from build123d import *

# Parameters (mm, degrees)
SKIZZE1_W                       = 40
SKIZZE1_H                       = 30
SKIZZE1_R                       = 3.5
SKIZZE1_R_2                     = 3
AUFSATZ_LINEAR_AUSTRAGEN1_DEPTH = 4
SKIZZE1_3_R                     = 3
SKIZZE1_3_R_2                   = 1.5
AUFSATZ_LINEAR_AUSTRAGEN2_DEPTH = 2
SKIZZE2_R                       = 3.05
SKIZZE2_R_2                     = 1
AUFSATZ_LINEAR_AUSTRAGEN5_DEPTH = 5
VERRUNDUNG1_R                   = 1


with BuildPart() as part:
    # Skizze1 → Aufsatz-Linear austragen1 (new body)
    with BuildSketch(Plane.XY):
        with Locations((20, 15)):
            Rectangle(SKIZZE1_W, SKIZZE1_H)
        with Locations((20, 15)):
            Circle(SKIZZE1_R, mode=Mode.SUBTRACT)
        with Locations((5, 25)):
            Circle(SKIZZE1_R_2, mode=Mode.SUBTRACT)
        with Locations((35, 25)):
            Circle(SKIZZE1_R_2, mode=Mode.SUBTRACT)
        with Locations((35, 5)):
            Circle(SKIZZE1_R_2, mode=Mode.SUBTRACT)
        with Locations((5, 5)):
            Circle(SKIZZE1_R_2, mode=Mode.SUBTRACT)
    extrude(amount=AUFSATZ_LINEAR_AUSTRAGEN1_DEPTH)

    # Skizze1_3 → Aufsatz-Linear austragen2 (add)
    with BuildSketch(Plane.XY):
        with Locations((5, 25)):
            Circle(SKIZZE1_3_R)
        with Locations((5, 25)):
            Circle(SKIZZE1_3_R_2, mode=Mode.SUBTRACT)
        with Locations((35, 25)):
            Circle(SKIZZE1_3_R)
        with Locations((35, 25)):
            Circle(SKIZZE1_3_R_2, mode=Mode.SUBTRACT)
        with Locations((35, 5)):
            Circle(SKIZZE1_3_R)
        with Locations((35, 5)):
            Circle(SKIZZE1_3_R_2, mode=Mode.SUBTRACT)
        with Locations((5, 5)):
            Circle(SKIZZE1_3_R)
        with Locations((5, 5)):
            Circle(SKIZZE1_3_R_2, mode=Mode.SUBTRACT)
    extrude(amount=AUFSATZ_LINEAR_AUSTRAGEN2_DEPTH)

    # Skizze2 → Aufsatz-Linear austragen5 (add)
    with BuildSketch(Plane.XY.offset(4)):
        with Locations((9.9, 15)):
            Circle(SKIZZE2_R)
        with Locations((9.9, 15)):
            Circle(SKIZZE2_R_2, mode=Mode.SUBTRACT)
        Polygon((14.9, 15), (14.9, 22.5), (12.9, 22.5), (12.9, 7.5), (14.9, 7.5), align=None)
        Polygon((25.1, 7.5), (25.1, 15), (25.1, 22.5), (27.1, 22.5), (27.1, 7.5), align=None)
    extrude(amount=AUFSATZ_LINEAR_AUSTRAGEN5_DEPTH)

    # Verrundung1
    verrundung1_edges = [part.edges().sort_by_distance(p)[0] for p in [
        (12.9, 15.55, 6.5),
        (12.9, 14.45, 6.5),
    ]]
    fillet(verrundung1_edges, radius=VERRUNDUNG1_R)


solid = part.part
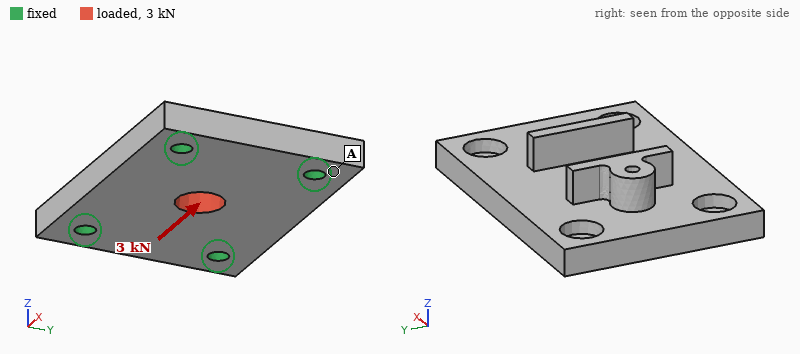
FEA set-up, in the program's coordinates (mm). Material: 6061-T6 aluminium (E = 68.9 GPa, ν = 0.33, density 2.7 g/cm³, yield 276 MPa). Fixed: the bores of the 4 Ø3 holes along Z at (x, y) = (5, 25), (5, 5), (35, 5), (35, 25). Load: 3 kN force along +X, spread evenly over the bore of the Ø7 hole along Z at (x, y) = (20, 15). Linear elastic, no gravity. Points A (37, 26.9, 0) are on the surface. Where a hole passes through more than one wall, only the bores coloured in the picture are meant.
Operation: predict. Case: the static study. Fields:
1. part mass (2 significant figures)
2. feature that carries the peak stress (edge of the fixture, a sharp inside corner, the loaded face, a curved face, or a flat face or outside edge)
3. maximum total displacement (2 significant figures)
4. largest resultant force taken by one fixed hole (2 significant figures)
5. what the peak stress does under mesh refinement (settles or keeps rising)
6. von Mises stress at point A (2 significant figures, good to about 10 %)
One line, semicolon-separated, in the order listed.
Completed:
13 g; edge of the fixture; 7.3 µm; 780 N; keeps rising; 14 MPa
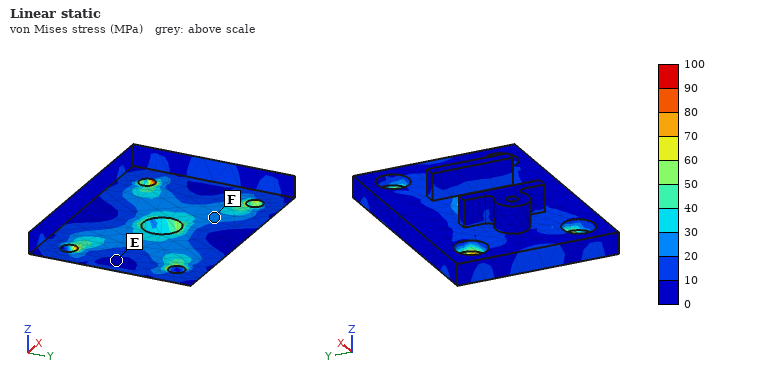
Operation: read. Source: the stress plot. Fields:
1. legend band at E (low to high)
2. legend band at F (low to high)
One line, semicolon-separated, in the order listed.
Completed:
0 to 10 MPa; 20 to 30 MPa
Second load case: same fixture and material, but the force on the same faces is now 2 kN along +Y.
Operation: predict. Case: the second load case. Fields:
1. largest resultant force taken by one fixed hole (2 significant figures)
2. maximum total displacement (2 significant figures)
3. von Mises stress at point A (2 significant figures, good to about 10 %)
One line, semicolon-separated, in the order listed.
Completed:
570 N; 7.3 µm; 12 MPa
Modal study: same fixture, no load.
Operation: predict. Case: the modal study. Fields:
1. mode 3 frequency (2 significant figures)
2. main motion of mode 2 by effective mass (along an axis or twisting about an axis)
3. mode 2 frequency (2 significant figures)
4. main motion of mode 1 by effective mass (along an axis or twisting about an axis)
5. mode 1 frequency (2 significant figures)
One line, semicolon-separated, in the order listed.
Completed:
31 kHz; twisting about X; 20 kHz; along Z; 14 kHz
